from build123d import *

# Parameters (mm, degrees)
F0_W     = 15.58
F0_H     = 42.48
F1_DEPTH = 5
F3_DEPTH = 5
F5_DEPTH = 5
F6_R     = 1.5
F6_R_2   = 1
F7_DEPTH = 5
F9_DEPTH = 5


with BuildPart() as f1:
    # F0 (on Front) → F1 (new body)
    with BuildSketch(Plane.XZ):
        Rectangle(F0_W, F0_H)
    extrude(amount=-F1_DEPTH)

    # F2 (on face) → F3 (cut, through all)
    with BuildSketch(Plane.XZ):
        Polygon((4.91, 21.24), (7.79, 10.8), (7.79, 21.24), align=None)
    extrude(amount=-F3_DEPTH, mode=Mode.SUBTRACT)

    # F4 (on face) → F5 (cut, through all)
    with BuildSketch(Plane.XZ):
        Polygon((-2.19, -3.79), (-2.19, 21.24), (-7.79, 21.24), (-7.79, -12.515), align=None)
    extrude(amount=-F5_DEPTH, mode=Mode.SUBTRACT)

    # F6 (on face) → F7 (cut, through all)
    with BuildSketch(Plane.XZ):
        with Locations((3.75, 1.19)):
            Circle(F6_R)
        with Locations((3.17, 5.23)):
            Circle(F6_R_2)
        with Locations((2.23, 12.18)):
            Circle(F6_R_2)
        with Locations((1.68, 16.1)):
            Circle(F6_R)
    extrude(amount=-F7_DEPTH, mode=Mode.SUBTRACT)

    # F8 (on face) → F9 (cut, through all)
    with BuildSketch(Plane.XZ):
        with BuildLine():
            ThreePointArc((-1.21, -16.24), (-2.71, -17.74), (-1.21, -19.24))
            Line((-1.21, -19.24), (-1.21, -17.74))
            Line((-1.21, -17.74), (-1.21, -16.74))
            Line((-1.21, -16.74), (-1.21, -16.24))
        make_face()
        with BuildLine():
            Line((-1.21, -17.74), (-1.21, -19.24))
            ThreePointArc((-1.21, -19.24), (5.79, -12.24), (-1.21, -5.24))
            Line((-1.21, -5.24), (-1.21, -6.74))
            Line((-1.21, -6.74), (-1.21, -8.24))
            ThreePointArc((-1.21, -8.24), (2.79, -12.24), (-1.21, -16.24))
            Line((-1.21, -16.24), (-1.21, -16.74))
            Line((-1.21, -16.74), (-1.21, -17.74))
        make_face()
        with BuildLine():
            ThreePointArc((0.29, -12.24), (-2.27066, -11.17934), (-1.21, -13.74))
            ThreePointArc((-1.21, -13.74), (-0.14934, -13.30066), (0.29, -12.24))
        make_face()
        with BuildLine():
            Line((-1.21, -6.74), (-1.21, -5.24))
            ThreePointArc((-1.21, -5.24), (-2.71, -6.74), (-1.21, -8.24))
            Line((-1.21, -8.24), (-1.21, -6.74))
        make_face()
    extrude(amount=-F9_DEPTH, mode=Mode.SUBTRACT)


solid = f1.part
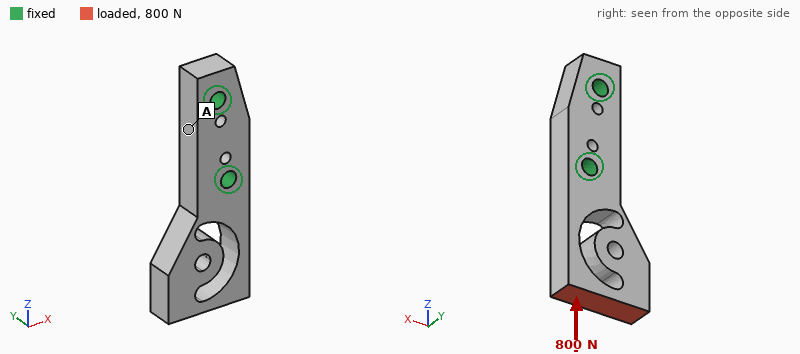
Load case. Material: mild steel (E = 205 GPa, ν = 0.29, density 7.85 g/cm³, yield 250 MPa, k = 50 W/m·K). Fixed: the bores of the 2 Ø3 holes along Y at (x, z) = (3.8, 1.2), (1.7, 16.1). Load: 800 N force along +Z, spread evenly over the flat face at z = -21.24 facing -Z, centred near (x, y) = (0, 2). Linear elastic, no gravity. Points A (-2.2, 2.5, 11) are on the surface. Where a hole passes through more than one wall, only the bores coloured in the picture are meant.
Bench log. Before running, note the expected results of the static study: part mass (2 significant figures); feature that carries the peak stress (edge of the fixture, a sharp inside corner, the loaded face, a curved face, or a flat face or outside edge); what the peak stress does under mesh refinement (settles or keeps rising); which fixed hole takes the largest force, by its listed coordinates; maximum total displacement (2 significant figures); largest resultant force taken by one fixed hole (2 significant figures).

16 g
a sharp inside corner
keeps rising
(3.8, 1.2)
23 µm
660 N
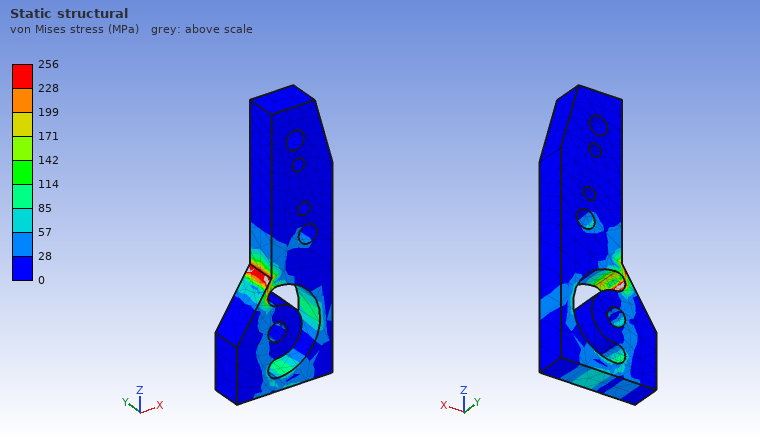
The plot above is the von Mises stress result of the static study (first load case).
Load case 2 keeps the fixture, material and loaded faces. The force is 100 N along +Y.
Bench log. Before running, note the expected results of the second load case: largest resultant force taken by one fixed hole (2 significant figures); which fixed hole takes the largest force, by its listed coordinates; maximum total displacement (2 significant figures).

130 N
(3.8, 1.2)
38 µm
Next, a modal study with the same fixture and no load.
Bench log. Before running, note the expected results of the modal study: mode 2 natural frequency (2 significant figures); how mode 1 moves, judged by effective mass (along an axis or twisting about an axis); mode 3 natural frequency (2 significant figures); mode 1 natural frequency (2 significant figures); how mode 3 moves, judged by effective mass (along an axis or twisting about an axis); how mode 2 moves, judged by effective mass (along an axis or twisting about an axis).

6800 Hz
along Y
12 kHz
5300 Hz
twisting about Z
along X
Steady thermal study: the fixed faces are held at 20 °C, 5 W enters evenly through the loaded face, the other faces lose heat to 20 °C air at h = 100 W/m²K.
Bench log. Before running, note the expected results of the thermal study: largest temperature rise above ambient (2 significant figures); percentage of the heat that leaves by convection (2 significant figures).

47 K
47 %
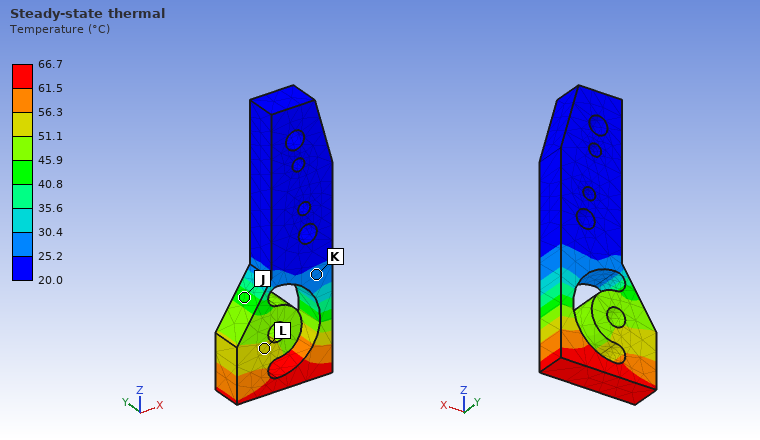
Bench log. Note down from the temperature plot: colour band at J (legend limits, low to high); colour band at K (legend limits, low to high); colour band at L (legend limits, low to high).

40.8 to 45.9 °C
25.2 to 30.4 °C
51.1 to 56.3 °C
